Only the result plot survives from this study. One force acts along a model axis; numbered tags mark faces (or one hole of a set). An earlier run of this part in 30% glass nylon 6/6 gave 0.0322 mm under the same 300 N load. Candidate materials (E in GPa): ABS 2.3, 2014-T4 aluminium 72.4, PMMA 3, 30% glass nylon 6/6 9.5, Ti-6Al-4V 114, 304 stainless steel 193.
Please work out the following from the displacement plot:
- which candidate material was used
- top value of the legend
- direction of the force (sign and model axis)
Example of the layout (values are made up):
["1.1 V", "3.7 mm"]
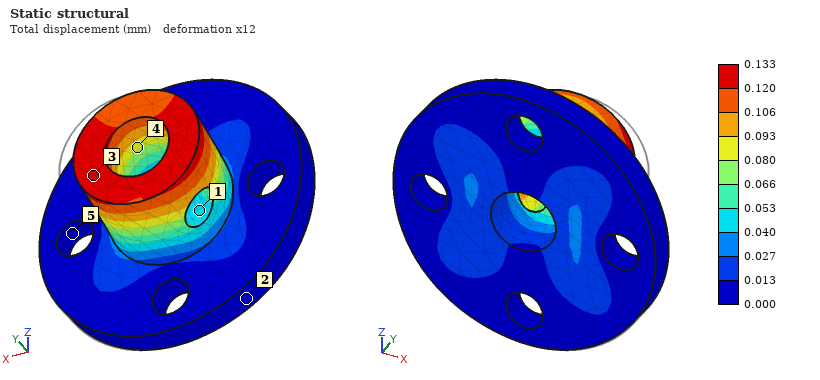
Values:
["ABS", "0.133 mm", "-X"]
